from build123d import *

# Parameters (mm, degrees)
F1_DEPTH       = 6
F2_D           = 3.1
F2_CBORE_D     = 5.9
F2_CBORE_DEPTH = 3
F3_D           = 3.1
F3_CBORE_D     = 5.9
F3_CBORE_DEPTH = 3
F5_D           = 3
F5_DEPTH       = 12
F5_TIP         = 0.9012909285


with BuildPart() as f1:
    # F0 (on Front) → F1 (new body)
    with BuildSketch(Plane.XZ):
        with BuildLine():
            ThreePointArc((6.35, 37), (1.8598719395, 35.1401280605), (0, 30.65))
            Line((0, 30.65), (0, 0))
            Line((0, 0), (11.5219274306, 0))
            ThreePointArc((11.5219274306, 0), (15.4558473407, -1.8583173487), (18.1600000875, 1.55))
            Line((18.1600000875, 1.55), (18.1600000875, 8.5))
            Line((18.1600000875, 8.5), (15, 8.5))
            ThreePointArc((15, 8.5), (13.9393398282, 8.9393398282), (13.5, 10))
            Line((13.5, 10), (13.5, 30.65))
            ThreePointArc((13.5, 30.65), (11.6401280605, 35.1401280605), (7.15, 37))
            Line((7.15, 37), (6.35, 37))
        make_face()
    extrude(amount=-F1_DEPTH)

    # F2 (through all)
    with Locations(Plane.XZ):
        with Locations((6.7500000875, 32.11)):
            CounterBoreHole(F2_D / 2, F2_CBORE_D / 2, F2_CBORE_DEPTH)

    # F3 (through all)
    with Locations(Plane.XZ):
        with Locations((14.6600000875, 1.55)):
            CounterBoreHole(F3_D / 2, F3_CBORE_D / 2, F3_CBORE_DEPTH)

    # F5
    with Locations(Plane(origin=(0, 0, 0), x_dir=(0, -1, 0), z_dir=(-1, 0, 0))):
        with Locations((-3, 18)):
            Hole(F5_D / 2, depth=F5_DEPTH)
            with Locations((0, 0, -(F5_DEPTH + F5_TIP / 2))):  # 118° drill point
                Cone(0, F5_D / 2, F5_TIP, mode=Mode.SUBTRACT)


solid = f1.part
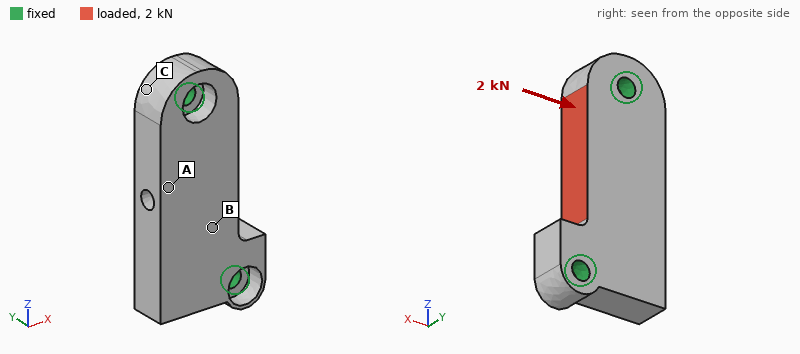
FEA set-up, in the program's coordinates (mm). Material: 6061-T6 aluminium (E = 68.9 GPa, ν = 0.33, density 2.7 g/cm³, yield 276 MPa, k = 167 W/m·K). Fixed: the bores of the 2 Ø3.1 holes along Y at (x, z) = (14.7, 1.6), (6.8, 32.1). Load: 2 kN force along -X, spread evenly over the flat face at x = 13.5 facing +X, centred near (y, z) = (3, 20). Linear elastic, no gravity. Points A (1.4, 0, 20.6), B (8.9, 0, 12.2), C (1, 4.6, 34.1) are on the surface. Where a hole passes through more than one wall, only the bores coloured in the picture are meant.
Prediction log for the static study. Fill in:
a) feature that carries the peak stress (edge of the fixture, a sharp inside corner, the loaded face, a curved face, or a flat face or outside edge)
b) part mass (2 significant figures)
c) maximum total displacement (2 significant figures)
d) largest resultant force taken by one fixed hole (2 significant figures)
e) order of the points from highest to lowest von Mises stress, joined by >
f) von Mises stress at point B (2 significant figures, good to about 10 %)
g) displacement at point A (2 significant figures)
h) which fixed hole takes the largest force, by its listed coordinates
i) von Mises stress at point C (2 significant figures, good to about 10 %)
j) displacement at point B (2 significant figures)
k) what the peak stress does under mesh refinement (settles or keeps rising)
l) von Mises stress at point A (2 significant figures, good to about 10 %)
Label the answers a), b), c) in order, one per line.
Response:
a) edge of the fixture
b) 7.8 g
c) 24 µm
d) 1.2 kN
e) A > B > C
f) 23 MPa
g) 21 µm
h) (6.8, 32.1)
i) 12 MPa
j) 18 µm
k) keeps rising
l) 45 MPa
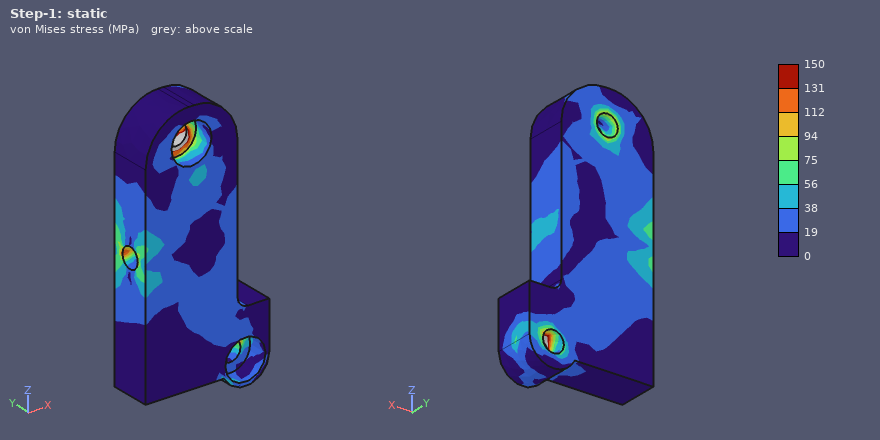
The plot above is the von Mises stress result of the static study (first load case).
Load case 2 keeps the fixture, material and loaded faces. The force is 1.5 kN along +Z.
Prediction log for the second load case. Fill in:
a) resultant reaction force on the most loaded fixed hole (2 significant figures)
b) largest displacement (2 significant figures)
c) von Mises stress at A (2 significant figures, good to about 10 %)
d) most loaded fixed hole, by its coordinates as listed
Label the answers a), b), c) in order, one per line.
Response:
a) 1.1 kN
b) 8.4 µm
c) 12 MPa
d) (6.8, 32.1)
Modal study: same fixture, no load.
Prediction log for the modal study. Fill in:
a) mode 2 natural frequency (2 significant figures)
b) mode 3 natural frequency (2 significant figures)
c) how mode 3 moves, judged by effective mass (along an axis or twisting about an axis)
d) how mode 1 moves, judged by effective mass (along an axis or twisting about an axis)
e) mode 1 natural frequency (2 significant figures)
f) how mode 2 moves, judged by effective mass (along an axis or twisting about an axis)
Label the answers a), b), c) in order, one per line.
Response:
a) 24 kHz
b) 27 kHz
c) along X
d) along Y
e) 12 kHz
f) along Y
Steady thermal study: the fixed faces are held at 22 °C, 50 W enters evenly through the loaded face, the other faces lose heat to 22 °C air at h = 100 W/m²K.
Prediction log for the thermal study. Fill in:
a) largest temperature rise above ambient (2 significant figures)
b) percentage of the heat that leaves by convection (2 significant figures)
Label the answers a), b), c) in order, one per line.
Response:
a) 37 K
b) 5.4 %
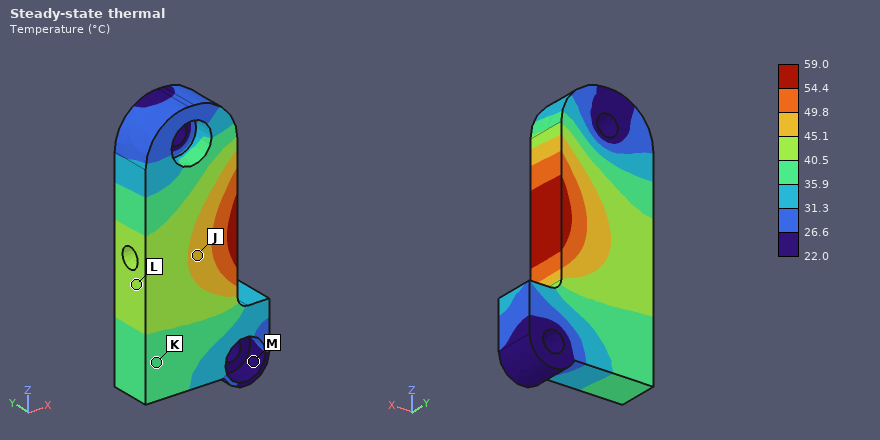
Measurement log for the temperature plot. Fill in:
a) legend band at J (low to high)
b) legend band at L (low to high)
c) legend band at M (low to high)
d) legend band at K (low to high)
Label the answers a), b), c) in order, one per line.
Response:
a) 45.1 to 49.8 °C
b) 40.5 to 45.1 °C
c) 22.0 to 26.6 °C
d) 35.9 to 40.5 °C
